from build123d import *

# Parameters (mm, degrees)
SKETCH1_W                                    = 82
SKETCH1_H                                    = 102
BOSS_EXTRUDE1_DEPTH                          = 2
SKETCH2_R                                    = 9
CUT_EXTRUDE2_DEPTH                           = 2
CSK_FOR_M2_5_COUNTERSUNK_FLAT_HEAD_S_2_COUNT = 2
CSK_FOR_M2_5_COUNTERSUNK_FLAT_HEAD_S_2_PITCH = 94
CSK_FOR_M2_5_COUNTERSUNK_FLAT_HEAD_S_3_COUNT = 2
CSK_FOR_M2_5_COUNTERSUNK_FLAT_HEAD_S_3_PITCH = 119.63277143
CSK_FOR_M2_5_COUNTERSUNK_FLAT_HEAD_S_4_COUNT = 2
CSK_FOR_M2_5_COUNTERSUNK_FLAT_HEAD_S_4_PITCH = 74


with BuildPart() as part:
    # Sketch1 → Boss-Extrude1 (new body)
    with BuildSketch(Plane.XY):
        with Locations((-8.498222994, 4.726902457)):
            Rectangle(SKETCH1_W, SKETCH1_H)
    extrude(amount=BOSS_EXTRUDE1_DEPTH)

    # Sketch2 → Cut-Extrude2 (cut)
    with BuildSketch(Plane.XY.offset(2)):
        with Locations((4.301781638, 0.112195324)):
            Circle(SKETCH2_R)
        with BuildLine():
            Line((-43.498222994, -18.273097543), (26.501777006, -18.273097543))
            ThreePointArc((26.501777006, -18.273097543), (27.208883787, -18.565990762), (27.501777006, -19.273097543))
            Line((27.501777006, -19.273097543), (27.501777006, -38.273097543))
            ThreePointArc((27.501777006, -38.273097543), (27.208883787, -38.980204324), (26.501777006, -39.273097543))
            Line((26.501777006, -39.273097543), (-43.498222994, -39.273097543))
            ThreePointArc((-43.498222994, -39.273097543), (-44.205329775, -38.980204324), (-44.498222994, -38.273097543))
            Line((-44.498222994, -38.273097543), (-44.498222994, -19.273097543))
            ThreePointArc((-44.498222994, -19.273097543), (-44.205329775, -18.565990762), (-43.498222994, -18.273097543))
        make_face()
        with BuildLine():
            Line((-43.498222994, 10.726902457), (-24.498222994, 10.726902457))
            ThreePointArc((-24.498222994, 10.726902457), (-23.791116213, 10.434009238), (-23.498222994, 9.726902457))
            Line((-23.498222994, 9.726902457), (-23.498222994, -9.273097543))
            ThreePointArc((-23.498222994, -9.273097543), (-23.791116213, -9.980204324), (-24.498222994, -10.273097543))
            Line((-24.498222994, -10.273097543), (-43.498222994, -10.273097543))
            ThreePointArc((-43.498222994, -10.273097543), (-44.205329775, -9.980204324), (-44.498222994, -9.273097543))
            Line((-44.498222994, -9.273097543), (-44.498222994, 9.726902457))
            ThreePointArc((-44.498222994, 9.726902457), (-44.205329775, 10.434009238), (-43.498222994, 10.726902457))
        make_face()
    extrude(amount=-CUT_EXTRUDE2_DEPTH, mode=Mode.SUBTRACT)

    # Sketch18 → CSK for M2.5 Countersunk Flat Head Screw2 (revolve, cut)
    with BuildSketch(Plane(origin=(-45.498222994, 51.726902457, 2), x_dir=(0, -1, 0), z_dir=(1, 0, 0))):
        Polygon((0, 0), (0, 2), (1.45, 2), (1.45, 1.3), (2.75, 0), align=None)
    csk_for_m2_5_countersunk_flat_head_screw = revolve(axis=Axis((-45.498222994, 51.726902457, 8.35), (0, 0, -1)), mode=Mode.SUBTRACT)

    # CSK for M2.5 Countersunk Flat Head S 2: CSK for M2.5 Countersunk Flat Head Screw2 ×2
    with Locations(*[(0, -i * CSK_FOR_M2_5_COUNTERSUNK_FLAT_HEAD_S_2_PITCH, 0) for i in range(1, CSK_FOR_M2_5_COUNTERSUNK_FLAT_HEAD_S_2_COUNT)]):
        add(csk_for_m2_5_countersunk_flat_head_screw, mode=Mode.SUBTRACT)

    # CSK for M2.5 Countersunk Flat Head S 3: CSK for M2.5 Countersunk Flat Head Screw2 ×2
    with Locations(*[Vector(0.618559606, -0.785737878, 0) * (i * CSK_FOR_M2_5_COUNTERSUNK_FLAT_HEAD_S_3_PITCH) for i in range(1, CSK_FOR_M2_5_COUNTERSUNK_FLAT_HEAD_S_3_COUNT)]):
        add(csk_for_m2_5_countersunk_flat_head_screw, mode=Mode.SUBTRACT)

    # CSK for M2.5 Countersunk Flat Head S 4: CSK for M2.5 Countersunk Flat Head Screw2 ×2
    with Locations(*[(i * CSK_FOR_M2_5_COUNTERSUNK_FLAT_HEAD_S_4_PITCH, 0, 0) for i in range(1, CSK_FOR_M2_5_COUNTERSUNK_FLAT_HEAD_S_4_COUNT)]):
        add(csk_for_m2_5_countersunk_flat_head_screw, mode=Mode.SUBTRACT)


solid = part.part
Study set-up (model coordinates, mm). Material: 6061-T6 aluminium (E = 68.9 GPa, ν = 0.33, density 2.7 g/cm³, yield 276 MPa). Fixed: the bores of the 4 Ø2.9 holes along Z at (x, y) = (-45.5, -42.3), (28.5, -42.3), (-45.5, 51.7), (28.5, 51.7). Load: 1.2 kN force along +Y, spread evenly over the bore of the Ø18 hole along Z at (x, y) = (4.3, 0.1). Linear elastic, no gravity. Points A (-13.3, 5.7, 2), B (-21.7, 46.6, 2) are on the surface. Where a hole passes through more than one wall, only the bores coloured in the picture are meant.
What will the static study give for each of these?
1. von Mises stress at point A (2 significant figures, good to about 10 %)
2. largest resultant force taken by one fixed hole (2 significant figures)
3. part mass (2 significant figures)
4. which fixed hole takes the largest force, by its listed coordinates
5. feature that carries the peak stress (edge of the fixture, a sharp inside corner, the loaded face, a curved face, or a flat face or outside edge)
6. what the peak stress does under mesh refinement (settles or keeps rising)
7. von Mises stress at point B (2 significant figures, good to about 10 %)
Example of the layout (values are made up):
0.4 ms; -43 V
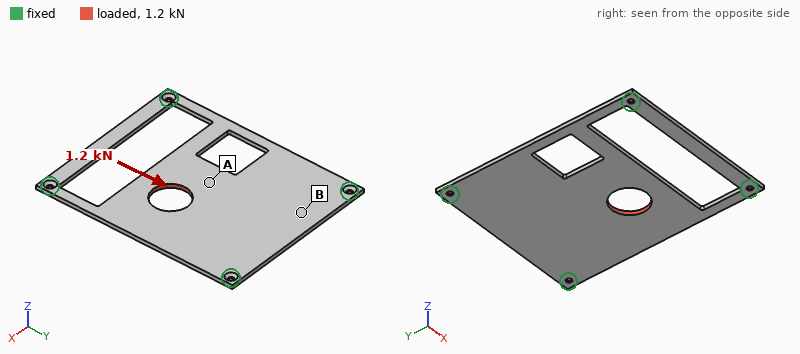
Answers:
13 MPa; 640 N; 33 g; (28.5, 51.7); edge of the fixture; keeps rising; 4.2 MPa
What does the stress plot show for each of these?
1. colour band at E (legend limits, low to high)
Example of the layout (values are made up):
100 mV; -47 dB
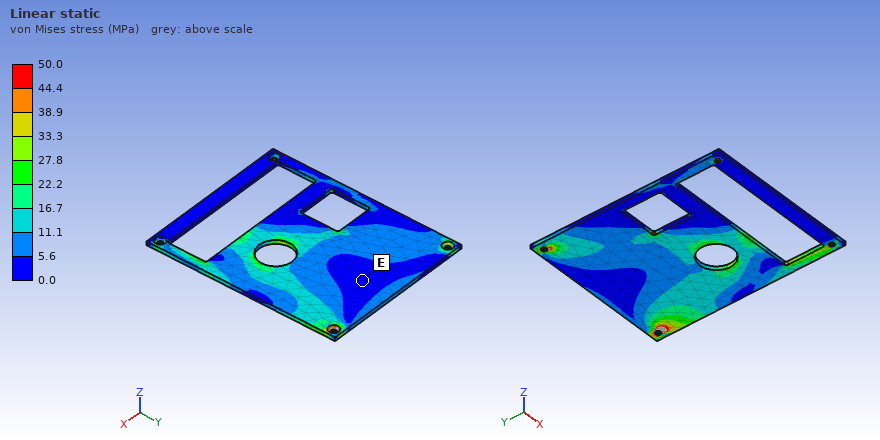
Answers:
0.0 to 5.6 MPa
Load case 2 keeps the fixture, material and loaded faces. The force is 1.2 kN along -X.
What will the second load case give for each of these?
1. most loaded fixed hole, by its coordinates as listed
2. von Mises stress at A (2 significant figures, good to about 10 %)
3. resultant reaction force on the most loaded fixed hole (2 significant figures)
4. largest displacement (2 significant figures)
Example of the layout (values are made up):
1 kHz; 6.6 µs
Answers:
(-45.5, 51.7); 21 MPa; 890 N; 47 µm
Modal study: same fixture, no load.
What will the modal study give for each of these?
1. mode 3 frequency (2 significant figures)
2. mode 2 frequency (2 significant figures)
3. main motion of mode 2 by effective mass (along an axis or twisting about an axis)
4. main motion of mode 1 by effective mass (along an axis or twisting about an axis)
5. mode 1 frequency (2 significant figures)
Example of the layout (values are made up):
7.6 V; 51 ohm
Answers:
1600 Hz; 1200 Hz; twisting about Y; along Z; 620 Hz
